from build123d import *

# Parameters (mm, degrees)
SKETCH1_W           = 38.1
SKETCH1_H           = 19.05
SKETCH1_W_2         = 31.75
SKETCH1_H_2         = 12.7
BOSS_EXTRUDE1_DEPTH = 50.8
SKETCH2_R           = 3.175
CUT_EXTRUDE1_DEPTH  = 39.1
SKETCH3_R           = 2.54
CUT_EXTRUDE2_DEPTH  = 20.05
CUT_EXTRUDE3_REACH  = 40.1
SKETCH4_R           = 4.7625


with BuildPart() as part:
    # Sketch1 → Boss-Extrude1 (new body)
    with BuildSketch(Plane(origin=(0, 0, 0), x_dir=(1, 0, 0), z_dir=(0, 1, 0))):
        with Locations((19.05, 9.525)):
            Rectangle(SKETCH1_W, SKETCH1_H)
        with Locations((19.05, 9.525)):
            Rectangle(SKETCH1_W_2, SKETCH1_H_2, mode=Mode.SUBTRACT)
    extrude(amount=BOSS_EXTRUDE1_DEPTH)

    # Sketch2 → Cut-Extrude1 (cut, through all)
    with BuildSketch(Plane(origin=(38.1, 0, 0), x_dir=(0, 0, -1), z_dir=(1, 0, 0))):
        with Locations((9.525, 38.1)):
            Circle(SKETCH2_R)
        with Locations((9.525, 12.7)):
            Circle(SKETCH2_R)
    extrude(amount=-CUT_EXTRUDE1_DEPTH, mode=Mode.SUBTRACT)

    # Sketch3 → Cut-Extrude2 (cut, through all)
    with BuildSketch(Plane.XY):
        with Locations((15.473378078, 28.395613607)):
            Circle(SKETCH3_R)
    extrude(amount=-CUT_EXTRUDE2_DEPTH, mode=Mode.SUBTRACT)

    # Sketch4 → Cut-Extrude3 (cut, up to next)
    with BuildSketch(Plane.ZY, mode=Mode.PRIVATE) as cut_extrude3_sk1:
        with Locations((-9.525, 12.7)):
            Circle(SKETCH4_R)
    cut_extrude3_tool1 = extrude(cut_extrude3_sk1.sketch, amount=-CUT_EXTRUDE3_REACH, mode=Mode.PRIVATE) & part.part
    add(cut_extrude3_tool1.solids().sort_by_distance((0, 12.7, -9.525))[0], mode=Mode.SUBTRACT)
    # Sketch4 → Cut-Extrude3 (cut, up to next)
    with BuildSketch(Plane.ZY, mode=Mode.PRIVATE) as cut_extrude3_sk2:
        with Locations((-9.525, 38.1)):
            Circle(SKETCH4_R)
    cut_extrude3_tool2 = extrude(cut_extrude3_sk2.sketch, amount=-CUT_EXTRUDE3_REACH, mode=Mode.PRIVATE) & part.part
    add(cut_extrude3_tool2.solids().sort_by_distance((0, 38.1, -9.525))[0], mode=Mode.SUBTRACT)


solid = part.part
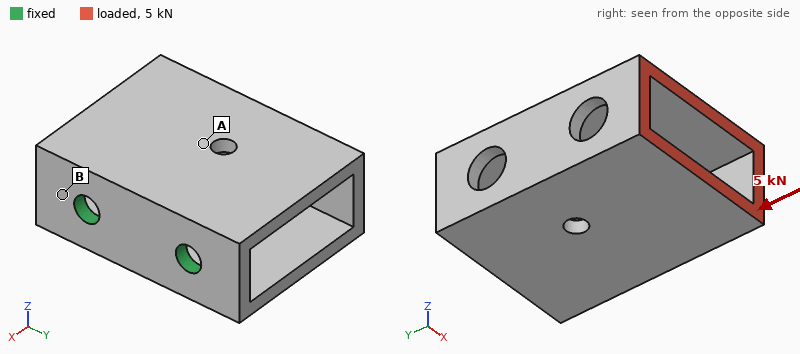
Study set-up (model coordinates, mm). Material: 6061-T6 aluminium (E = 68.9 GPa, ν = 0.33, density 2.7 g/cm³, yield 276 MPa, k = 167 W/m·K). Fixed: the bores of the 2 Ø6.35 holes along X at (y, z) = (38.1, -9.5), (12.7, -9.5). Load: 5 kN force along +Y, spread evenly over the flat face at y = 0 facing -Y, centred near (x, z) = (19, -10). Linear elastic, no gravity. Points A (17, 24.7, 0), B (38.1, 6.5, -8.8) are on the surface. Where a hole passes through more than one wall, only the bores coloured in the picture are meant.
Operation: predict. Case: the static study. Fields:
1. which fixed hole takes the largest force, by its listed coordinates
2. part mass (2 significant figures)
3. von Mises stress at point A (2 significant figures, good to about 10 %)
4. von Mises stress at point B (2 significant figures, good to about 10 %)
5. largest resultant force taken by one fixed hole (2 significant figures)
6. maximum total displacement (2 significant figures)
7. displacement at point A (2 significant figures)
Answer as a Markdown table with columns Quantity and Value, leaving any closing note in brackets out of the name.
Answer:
| Quantity | Value |
|---|---|
| which fixed hole takes the largest force, by its listed coordinates | (12.7, -9.5) |
| part mass | 42 g |
| von Mises stress at point A | 45 MPa |
| von Mises stress at point B | 120 MPa |
| largest resultant force taken by one fixed hole | 4.2 kN |
| maximum total displacement | 0.12 mm |
| displacement at point A | 0.051 mm |
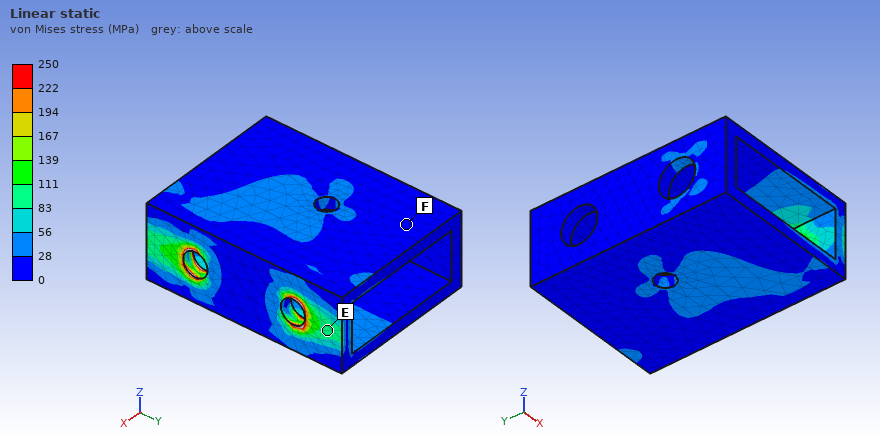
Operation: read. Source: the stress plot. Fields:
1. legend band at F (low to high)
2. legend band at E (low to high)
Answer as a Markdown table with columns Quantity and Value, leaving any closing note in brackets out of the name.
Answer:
| Quantity | Value |
|---|---|
| legend band at F | 0 to 28 MPa |
| legend band at E | 83 to 111 MPa |
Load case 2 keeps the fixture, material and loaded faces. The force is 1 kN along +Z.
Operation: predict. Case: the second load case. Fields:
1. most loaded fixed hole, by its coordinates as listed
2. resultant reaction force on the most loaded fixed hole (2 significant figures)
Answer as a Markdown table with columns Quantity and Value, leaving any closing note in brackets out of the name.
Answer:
| Quantity | Value |
|---|---|
| most loaded fixed hole, by its coordinates as listed | (12.7, -9.5) |
| resultant reaction force on the most loaded fixed hole | 1.3 kN |
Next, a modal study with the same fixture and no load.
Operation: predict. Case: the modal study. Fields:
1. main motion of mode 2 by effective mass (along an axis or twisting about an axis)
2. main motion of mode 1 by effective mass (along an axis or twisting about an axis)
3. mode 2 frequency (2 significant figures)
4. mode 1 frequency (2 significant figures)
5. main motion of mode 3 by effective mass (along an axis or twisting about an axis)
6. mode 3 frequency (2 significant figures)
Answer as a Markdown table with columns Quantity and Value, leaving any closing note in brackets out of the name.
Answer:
| Quantity | Value |
|---|---|
| main motion of mode 2 by effective mass | twisting about X |
| main motion of mode 1 by effective mass | along Z |
| mode 2 frequency | 5200 Hz |
| mode 1 frequency | 1800 Hz |
| main motion of mode 3 by effective mass | along Y |
| mode 3 frequency | 5700 Hz |
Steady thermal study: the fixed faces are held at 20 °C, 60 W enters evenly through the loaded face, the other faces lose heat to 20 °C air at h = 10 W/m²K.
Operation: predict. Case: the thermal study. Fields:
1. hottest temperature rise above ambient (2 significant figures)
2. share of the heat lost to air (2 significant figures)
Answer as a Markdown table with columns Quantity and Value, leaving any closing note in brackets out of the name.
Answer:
| Quantity | Value |
|---|---|
| hottest temperature rise above ambient | 49 K |
| share of the heat lost to air | 3.4 % |
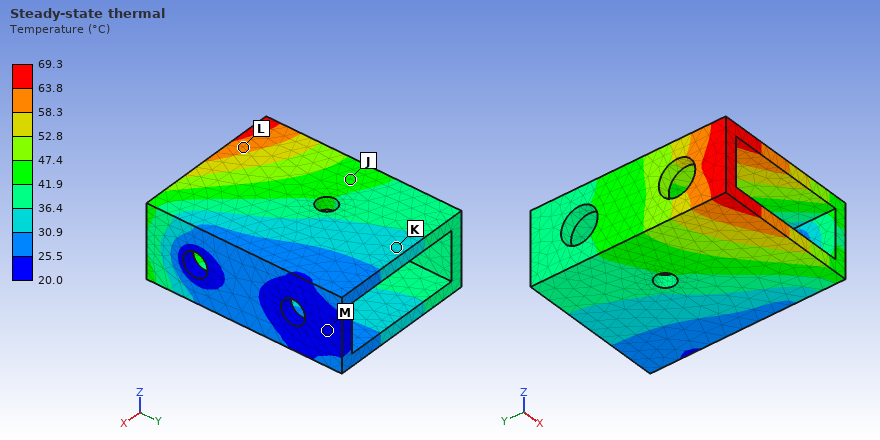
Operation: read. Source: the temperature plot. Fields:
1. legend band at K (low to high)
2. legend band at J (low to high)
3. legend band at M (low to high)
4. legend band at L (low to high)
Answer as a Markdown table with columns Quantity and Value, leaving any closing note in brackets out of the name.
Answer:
| Quantity | Value |
|---|---|
| legend band at K | 30.9 to 36.4 °C |
| legend band at J | 41.9 to 47.4 °C |
| legend band at M | 20.0 to 25.5 °C |
| legend band at L | 58.3 to 63.8 °C |
